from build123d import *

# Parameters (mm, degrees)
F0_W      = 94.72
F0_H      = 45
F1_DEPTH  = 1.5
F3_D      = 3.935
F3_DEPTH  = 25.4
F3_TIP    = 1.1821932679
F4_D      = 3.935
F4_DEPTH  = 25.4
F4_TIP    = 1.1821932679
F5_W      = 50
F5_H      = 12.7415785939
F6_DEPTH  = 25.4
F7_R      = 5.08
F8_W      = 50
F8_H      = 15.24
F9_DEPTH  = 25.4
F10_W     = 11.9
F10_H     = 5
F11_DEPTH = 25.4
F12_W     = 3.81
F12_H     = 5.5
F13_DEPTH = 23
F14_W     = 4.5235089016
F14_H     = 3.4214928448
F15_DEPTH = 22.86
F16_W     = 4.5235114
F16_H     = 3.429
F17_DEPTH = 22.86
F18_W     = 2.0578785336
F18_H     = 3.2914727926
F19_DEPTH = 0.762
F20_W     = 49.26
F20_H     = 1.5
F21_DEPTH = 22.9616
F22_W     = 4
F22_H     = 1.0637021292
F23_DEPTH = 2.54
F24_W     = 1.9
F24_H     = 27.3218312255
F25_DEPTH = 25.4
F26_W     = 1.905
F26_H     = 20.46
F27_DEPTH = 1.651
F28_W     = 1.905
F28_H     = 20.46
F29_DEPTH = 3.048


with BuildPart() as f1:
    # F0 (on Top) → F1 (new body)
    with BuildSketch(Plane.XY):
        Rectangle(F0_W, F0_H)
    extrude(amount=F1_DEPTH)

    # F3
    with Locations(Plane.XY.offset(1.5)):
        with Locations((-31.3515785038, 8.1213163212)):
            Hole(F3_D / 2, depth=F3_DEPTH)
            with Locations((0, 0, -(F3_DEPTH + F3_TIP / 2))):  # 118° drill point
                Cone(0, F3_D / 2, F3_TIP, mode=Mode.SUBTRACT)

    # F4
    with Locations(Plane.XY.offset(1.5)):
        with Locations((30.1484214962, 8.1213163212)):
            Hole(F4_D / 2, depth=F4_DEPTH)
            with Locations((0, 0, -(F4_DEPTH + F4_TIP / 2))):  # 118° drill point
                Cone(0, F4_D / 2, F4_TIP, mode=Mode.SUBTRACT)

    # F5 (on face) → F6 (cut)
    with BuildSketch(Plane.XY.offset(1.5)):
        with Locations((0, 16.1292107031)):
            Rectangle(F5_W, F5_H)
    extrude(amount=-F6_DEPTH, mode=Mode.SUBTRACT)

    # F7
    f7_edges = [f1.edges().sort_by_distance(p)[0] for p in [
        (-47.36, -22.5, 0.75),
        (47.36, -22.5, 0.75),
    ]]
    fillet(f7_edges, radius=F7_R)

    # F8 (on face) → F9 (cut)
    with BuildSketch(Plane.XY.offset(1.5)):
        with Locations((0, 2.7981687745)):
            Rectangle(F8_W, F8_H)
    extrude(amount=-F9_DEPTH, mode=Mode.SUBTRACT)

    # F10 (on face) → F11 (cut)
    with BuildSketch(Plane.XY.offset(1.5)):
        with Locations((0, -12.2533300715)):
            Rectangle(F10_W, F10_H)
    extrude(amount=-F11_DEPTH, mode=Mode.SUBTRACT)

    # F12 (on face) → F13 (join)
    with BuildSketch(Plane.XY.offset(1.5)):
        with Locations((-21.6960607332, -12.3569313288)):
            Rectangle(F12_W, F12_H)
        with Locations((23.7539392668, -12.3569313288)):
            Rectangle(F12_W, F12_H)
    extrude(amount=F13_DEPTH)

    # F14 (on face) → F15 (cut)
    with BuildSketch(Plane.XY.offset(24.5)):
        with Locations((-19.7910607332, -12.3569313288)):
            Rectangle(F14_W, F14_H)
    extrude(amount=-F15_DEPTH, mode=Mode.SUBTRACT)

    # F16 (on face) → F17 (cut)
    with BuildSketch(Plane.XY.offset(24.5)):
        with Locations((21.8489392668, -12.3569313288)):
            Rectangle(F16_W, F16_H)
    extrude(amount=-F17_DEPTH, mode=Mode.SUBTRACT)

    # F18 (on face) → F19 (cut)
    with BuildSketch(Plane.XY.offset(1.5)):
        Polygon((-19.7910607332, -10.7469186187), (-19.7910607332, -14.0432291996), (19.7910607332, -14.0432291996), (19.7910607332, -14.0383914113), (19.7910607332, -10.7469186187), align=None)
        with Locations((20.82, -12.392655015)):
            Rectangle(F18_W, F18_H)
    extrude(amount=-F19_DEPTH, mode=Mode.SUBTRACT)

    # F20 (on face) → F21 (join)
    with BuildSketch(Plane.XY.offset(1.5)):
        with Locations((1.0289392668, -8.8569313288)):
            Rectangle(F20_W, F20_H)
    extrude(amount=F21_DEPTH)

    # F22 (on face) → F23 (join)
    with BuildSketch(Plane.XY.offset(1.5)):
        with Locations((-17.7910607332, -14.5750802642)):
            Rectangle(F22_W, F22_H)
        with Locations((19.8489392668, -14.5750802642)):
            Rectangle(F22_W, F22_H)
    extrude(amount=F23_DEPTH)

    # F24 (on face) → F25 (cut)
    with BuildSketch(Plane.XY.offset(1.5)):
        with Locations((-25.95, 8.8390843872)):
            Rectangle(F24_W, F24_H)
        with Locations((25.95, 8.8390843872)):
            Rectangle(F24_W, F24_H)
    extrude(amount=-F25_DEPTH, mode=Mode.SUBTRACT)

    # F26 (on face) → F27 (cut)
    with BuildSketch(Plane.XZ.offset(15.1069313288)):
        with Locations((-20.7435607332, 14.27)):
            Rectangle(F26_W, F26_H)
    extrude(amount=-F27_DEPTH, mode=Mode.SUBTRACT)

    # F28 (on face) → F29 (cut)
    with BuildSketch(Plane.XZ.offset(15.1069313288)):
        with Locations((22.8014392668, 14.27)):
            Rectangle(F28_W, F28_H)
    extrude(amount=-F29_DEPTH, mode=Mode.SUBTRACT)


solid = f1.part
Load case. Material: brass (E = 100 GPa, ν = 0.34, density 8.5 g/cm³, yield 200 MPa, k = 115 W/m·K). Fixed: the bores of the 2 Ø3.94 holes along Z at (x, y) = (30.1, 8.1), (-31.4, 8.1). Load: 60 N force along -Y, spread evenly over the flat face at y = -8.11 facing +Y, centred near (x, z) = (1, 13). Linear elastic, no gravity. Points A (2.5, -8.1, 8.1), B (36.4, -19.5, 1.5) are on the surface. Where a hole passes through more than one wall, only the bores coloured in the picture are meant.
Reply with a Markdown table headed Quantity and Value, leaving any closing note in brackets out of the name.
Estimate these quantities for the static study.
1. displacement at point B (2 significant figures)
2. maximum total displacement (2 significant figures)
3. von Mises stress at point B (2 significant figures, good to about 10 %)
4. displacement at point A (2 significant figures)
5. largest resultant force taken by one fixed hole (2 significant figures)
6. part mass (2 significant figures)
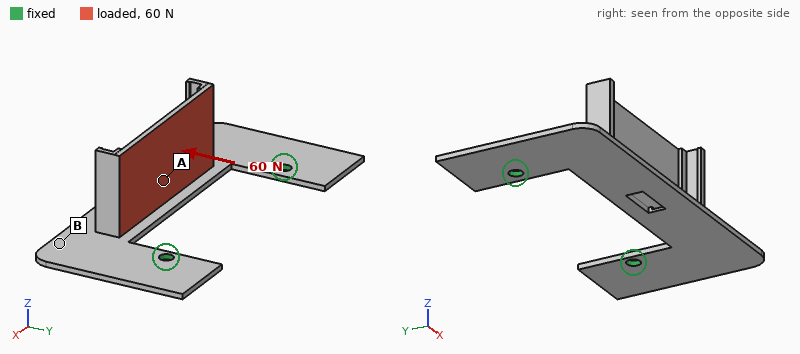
| Quantity | Value |
|---|---|
| displacement at point B | 0.23 mm |
| maximum total displacement | 0.41 mm |
| von Mises stress at point B | 14 MPa |
| displacement at point A | 0.15 mm |
| largest resultant force taken by one fixed hole | 34 N |
| part mass | 53 g |
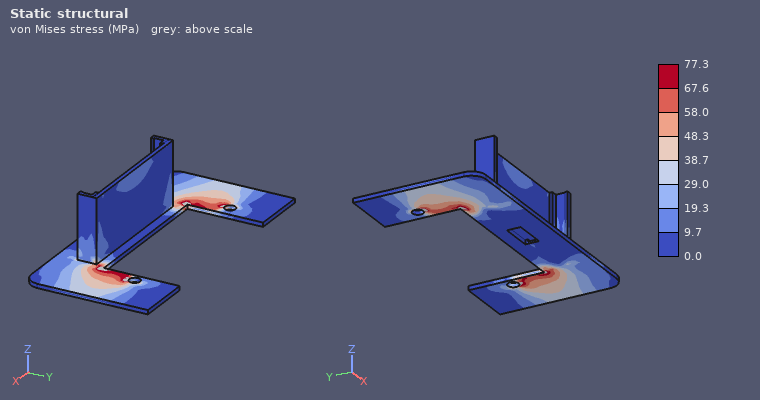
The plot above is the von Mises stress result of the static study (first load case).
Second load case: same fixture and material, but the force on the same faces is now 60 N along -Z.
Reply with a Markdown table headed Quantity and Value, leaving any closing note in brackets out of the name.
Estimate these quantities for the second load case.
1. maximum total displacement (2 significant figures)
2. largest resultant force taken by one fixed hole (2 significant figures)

| Quantity | Value |
|---|---|
| maximum total displacement | 0.21 mm |
| largest resultant force taken by one fixed hole | 31 N |
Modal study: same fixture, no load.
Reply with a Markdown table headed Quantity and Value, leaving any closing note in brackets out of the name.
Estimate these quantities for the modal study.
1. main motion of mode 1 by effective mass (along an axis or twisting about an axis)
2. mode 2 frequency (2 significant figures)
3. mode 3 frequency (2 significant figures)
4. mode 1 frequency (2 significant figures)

| Quantity | Value |
|---|---|
| main motion of mode 1 by effective mass | along Z |
| mode 2 frequency | 880 Hz |
| mode 3 frequency | 1200 Hz |
| mode 1 frequency | 380 Hz |
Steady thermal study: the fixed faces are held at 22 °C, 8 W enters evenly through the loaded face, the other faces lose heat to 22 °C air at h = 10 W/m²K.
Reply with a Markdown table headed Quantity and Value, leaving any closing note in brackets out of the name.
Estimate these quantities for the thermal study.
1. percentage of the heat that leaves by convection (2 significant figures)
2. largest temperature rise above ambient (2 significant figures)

| Quantity | Value |
|---|---|
| percentage of the heat that leaves by convection | 22 % |
| largest temperature rise above ambient | 42 K |
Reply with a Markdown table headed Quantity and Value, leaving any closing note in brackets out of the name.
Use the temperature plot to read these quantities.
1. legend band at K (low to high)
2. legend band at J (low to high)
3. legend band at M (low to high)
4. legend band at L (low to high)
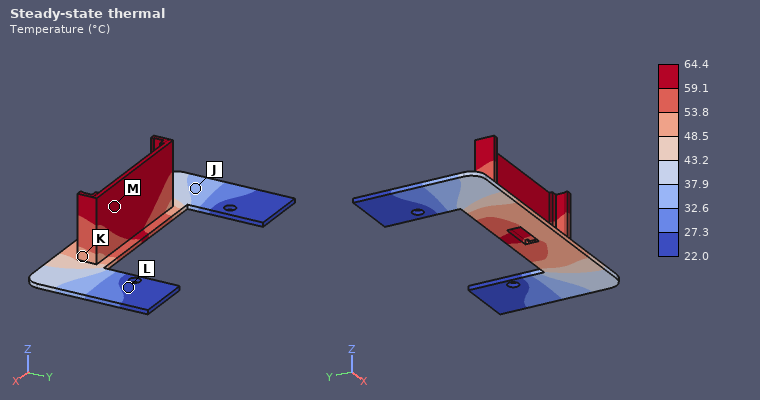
| Quantity | Value |
|---|---|
| legend band at K | 48.5 to 53.8 °C |
| legend band at J | 32.6 to 37.9 °C |
| legend band at M | 59.1 to 64.4 °C |
| legend band at L | 22.0 to 27.3 °C |
